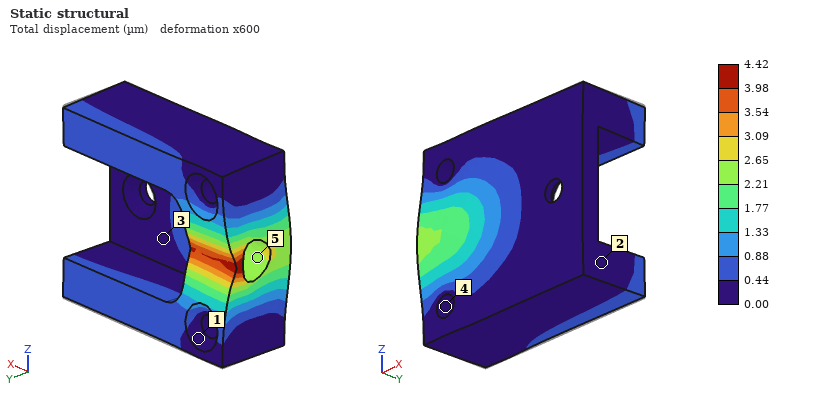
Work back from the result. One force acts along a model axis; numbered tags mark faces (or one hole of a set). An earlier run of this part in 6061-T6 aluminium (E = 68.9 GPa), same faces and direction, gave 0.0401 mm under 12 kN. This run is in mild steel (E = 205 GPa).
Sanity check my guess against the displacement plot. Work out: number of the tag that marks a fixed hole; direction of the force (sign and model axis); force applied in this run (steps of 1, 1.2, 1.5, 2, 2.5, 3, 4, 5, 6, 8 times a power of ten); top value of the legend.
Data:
4
-Y
4 kN
4.42 µm
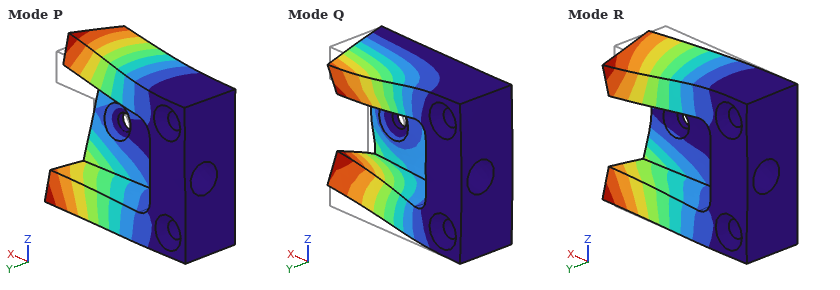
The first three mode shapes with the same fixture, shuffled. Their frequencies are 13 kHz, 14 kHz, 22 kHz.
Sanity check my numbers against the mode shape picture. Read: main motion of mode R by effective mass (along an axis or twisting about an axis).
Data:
along Y
